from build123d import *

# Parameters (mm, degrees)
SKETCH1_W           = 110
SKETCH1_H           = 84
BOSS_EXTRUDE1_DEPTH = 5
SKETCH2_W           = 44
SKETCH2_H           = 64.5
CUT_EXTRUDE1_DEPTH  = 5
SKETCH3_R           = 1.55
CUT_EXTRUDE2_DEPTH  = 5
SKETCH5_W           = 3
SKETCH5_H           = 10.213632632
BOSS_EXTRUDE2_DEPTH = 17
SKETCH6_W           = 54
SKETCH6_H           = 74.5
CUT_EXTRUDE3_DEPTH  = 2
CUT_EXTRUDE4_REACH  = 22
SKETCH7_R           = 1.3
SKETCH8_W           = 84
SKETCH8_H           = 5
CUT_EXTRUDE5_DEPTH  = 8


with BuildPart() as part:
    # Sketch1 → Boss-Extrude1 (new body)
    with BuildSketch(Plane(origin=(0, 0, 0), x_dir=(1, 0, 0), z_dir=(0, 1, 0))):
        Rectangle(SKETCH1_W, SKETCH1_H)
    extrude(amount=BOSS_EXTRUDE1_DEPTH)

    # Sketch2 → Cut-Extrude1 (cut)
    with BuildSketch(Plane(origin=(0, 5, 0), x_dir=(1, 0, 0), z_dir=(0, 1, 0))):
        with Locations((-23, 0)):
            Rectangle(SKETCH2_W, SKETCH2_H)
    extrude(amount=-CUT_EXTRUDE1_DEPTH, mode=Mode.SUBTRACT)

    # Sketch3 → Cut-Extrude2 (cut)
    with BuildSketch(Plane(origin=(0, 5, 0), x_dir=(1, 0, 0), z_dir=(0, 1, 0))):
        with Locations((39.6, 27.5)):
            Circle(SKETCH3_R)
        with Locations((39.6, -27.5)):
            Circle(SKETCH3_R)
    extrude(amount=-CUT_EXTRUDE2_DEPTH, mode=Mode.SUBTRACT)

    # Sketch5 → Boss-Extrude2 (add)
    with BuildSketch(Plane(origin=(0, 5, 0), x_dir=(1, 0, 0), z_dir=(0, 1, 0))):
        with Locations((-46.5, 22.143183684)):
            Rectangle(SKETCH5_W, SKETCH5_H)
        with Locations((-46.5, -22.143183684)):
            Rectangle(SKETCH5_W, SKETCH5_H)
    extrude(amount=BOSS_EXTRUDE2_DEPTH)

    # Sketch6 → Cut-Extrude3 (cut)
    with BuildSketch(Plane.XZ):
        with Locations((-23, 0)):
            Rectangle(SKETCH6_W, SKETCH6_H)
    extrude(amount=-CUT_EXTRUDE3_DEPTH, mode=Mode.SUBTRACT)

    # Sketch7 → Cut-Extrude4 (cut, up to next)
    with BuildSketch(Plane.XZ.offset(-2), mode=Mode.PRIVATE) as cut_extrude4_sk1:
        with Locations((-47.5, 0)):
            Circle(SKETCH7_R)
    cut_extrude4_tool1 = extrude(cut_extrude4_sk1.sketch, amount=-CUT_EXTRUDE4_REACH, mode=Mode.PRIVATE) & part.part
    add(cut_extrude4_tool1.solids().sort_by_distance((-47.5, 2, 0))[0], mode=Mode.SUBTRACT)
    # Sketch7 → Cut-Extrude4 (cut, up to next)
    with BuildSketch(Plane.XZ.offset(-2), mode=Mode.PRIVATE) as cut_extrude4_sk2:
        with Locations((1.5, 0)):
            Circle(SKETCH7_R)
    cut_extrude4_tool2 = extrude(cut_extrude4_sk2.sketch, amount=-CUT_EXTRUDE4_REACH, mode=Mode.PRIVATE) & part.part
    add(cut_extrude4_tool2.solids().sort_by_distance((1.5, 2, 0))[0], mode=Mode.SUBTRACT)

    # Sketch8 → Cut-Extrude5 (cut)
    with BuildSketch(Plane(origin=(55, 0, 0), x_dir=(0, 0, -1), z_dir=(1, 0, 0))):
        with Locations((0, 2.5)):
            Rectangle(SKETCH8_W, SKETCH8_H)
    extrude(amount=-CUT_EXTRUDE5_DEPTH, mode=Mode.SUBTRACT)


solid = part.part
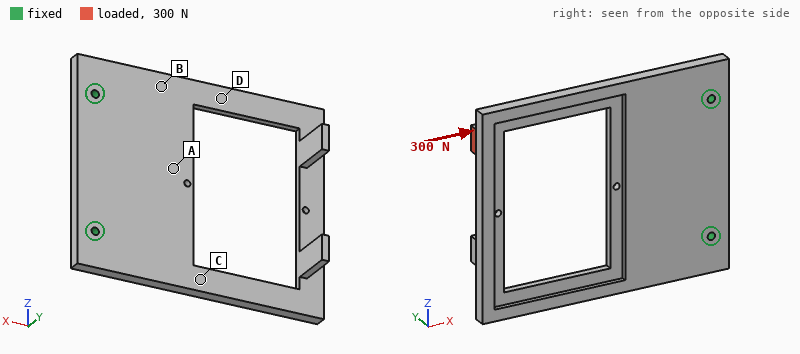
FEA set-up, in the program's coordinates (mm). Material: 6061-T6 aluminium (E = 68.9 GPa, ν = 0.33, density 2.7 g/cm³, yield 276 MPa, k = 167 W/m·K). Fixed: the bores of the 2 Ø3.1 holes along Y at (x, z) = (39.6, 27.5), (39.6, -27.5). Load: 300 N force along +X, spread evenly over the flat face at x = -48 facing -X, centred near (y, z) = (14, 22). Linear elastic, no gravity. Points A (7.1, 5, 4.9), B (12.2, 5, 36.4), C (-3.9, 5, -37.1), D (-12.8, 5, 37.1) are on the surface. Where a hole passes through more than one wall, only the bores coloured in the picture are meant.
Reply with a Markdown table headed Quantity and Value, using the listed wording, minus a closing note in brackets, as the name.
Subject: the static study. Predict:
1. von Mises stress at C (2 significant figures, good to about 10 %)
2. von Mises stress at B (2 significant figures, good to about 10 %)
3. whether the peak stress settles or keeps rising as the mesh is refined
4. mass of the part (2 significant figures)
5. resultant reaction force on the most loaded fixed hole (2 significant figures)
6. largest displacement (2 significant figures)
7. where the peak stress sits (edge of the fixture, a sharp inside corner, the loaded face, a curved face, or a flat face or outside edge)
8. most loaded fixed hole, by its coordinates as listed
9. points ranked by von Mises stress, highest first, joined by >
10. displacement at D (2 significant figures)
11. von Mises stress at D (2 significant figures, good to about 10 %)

| Quantity | Value |
|---|---|
| von Mises stress at C | 44 MPa |
| von Mises stress at B | 26 MPa |
| whether the peak stress settles or keeps rising as the mesh is refined | keeps rising |
| mass of the part | 73 g |
| resultant reaction force on the most loaded fixed hole | 270 N |
| largest displacement | 1.1 mm |
| where the peak stress sits | a sharp inside corner |
| most loaded fixed hole, by its coordinates as listed | (39.6, 27.5) |
| points ranked by von Mises stress, highest first, joined by > | D > C > B > A |
| displacement at D | 0.18 mm |
| von Mises stress at D | 65 MPa |
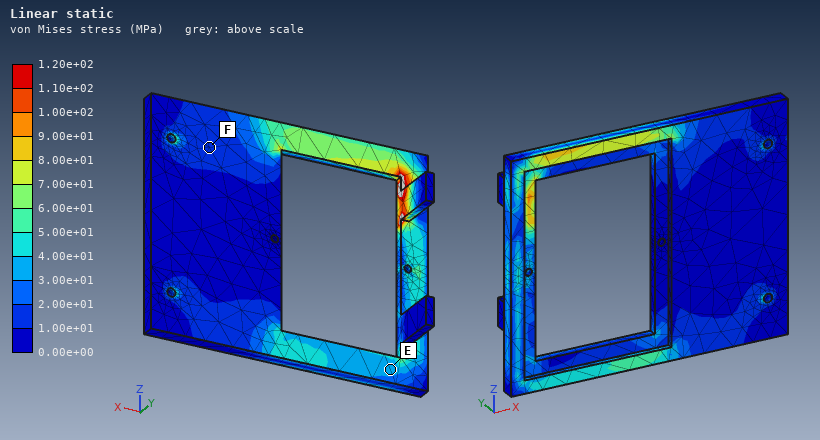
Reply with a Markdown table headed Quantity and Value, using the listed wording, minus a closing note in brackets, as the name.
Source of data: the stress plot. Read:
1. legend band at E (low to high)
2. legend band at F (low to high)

| Quantity | Value |
|---|---|
| legend band at E | 3.00e+01 to 4.00e+01 MPa |
| legend band at F | 1.00e+01 to 2.00e+01 MPa |
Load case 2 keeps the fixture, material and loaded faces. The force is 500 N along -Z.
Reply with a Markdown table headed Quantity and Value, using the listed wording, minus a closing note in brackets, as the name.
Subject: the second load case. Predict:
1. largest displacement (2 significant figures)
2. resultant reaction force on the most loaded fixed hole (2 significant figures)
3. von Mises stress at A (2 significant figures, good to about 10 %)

| Quantity | Value |
|---|---|
| largest displacement | 0.76 mm |
| resultant reaction force on the most loaded fixed hole | 820 N |
| von Mises stress at A | 21 MPa |
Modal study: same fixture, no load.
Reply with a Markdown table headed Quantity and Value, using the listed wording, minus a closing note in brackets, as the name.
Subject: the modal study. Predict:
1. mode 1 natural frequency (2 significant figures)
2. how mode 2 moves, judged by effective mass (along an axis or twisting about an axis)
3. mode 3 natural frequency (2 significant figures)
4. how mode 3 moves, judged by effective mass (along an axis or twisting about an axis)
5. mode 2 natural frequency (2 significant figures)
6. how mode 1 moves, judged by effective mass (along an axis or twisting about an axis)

| Quantity | Value |
|---|---|
| mode 1 natural frequency | 390 Hz |
| how mode 2 moves, judged by effective mass | twisting about X |
| mode 3 natural frequency | 1700 Hz |
| how mode 3 moves, judged by effective mass | along Z |
| mode 2 natural frequency | 830 Hz |
| how mode 1 moves, judged by effective mass | along Y |
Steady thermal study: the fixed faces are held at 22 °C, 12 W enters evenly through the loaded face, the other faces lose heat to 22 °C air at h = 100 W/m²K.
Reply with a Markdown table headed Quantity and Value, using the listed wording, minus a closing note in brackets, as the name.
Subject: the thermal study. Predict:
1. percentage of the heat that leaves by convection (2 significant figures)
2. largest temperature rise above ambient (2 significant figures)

| Quantity | Value |
|---|---|
| percentage of the heat that leaves by convection | 84 % |
| largest temperature rise above ambient | 54 K |
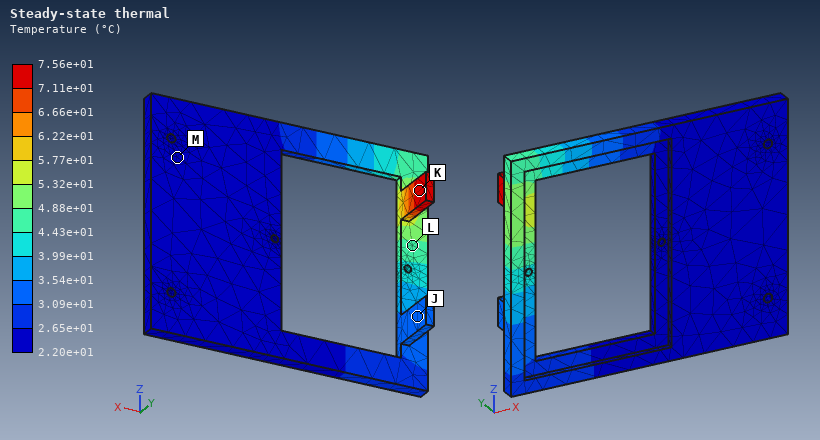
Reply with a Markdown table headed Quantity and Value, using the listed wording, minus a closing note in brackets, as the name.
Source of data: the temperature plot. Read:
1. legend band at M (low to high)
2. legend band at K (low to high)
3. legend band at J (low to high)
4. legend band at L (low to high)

| Quantity | Value |
|---|---|
| legend band at M | 2.20e+01 to 2.65e+01 °C |
| legend band at K | 7.11e+01 to 7.56e+01 °C |
| legend band at J | 3.09e+01 to 3.54e+01 °C |
| legend band at L | 4.43e+01 to 4.88e+01 °C |
